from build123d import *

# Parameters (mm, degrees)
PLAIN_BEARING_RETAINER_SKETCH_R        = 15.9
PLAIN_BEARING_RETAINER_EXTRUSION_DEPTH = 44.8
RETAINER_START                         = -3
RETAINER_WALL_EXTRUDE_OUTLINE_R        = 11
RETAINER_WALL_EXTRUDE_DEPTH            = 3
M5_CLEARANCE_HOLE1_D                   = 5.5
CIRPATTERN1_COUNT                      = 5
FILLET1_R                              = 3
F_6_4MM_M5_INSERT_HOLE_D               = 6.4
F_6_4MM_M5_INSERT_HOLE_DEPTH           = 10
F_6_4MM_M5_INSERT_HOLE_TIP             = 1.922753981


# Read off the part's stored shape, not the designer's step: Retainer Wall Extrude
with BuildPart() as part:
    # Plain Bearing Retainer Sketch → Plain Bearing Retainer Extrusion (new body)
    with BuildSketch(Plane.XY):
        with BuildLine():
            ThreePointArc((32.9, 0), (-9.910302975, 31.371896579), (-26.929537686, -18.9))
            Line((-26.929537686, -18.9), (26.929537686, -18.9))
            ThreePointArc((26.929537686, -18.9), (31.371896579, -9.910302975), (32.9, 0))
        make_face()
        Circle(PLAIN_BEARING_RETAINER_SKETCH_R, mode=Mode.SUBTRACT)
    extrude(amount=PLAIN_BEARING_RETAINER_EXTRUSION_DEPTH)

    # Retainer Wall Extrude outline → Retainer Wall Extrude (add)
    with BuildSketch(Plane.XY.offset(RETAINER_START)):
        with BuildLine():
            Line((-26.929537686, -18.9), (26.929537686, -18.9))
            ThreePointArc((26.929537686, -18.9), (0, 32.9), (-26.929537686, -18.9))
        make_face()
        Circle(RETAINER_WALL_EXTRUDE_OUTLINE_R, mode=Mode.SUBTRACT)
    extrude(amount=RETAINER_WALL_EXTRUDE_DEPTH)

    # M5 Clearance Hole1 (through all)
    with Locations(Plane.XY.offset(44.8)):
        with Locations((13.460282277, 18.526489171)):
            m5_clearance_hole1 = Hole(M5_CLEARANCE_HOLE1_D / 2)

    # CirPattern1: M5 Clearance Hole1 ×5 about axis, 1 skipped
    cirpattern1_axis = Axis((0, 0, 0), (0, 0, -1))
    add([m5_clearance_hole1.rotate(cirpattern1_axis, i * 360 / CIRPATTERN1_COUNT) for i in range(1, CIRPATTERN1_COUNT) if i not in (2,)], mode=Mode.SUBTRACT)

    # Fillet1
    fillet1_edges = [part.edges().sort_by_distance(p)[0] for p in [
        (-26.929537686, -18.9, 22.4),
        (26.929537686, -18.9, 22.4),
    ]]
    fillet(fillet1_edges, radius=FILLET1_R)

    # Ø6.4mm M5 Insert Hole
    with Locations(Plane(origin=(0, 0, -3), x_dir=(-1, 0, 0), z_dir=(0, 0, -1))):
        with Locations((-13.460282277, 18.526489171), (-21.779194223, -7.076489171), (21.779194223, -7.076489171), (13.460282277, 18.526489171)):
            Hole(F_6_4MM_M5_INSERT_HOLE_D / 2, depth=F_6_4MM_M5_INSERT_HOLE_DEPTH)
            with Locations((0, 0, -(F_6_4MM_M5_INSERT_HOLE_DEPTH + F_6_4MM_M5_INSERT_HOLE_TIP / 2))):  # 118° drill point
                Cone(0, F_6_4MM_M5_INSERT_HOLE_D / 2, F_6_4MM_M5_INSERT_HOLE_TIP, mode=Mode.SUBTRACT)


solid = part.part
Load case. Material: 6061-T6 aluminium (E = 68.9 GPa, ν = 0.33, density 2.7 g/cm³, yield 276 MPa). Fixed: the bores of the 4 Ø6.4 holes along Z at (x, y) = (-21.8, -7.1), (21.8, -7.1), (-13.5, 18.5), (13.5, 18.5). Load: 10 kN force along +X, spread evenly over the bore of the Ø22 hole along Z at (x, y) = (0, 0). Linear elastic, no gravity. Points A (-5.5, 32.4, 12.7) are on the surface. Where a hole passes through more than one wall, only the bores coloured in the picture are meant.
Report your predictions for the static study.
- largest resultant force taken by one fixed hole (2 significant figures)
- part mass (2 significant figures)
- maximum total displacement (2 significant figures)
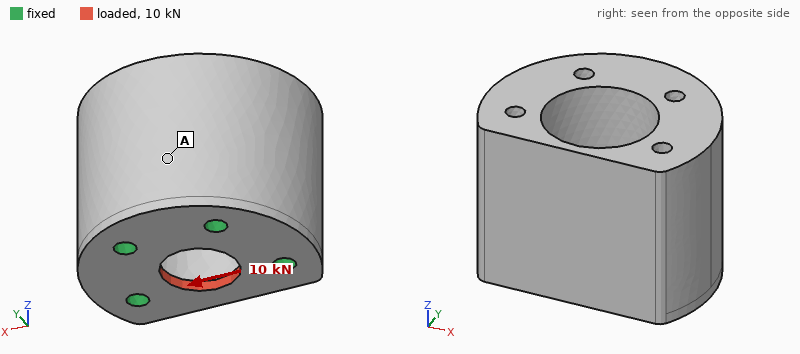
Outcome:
3.3 kN
260 g
12 µm
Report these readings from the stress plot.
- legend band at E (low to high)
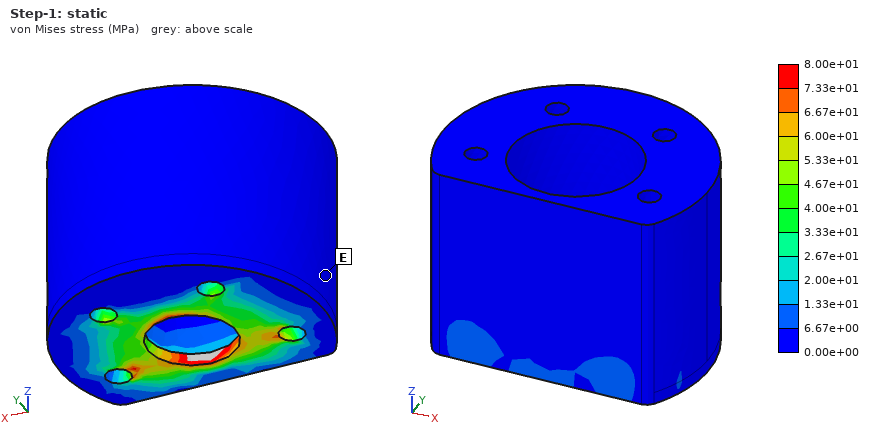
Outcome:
0.00e+00 to 6.67e+00 MPa
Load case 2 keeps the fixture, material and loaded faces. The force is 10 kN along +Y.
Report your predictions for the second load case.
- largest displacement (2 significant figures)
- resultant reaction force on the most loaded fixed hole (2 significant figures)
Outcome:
33 µm
2.7 kN
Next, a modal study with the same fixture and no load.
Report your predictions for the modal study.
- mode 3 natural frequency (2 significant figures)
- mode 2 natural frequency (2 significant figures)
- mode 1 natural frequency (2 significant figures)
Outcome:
15 kHz
9600 Hz
9300 Hz
